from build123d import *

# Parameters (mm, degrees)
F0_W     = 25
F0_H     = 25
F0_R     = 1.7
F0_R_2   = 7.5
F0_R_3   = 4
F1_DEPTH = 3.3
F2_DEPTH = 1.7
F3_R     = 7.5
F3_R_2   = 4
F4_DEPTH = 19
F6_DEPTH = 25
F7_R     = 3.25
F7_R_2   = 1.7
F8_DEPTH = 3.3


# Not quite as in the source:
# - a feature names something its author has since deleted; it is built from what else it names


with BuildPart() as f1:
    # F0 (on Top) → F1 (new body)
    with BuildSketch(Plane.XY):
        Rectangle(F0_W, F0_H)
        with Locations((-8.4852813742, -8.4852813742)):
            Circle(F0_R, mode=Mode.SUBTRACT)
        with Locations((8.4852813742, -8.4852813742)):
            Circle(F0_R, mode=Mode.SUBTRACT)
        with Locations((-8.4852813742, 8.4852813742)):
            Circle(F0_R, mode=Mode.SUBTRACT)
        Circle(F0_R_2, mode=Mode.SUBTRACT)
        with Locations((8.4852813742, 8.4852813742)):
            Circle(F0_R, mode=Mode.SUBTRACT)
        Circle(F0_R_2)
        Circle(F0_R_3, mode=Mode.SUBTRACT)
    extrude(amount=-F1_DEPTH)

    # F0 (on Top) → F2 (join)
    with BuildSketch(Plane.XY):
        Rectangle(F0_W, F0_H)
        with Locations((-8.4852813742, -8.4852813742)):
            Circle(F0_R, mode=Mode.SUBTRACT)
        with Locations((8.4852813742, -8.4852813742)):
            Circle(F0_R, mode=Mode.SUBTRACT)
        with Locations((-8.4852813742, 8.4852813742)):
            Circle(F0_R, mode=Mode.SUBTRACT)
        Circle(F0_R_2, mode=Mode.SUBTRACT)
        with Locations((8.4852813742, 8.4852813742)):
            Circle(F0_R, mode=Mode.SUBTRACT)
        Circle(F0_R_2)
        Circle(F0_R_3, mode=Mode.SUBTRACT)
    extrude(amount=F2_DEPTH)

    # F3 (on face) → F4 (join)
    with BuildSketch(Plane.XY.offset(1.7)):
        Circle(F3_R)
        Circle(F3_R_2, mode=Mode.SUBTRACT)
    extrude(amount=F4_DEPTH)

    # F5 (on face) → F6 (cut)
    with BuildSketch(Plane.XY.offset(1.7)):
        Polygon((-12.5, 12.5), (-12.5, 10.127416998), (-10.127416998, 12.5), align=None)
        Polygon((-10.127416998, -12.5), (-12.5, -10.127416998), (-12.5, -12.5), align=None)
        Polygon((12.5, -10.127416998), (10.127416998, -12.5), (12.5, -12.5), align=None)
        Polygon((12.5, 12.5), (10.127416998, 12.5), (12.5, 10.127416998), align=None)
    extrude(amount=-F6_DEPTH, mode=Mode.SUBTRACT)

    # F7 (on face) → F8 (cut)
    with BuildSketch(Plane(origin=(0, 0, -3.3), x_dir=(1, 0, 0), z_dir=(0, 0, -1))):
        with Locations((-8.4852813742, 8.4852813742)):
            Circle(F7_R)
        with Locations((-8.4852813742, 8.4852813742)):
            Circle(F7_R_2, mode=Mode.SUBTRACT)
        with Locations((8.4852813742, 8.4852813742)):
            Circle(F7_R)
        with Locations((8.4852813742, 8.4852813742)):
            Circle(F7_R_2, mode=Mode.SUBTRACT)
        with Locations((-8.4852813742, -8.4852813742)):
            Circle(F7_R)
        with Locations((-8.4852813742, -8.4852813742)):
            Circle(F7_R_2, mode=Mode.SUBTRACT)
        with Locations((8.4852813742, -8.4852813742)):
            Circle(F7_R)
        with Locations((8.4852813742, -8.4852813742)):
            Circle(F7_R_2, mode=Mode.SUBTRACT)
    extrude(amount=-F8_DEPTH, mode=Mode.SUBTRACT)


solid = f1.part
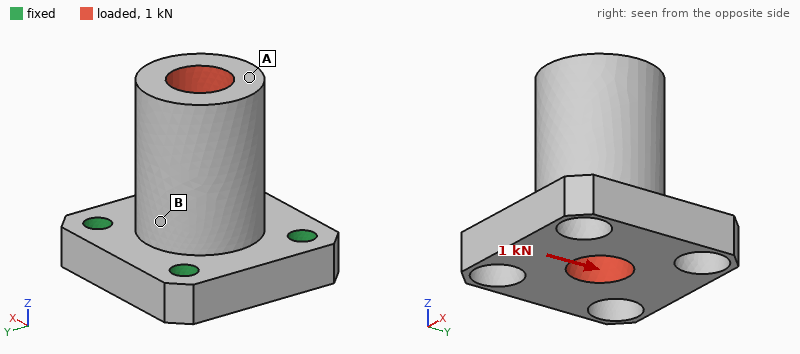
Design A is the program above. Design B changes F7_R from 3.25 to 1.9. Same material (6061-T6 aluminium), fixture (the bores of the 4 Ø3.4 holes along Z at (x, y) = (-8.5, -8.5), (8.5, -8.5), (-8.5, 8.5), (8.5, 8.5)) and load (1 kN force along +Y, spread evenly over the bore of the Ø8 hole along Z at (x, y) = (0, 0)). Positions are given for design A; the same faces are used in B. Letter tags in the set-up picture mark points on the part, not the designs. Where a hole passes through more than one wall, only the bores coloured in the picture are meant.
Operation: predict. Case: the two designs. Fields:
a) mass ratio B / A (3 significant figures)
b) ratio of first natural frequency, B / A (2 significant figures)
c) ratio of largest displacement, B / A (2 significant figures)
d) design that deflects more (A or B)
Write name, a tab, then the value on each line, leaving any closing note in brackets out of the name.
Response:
mass ratio B / A	1.06
ratio of first natural frequency, B / A	1.1
ratio of largest displacement, B / A	0.87
design that deflects more	A
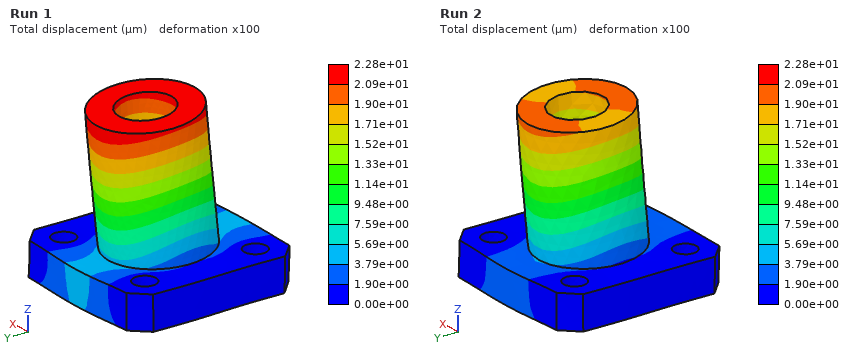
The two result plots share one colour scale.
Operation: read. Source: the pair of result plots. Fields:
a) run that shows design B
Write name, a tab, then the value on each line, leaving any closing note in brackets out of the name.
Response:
run that shows design B	Run 2
